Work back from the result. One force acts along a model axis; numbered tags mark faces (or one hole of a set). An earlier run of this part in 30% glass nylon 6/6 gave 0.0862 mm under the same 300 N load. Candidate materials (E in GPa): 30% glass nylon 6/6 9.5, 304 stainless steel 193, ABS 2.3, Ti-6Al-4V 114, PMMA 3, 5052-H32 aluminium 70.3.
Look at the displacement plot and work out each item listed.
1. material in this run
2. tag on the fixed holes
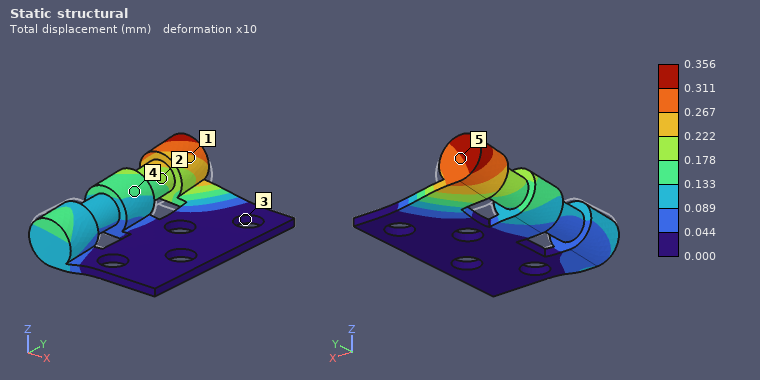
ABS
3
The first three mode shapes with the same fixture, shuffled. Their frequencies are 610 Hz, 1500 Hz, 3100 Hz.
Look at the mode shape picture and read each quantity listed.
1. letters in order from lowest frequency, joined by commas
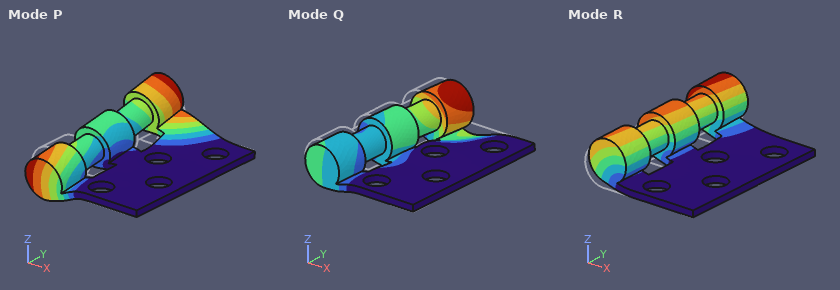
R, P, Q
